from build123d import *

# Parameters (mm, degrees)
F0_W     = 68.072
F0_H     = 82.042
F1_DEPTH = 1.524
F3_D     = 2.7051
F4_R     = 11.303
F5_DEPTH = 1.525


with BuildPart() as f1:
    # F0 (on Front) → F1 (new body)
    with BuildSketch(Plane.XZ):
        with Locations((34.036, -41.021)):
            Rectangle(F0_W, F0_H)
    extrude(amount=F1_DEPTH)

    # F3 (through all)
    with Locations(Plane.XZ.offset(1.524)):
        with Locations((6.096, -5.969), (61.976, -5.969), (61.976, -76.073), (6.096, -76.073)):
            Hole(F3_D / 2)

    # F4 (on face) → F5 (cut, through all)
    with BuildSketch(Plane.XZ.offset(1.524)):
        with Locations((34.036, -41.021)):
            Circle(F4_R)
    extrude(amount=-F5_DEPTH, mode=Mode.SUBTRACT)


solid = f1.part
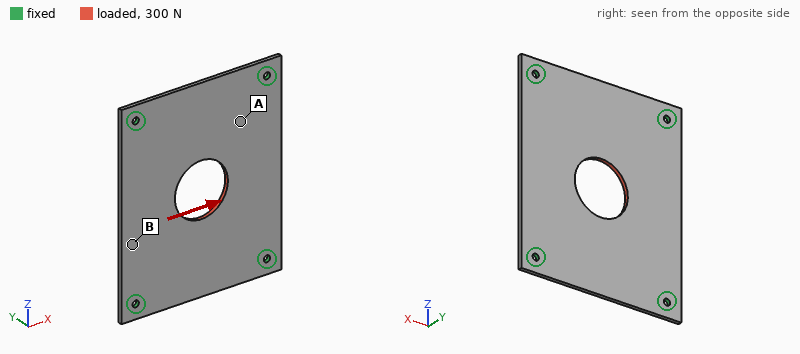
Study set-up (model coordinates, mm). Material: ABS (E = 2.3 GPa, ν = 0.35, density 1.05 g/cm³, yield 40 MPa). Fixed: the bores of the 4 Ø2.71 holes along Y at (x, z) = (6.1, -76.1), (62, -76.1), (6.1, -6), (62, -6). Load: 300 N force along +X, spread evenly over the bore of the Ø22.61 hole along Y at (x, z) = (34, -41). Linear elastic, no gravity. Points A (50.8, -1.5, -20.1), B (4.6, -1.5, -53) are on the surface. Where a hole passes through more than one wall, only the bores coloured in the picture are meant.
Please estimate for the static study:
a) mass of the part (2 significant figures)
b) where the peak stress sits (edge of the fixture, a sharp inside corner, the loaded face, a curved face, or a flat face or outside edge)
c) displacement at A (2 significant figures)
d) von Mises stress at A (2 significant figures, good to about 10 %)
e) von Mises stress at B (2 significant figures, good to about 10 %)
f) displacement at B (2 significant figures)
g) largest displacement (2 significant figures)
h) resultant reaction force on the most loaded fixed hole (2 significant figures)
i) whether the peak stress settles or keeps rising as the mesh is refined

8.3 g
edge of the fixture
44 µm
3.0 MPa
1.5 MPa
63 µm
85 µm
87 N
keeps rising
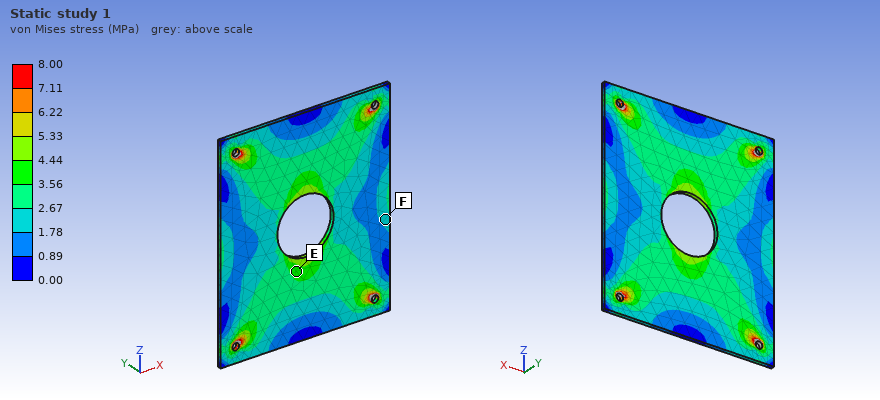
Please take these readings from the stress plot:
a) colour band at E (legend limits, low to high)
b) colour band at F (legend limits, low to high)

3.56 to 4.44 MPa
1.78 to 2.67 MPa
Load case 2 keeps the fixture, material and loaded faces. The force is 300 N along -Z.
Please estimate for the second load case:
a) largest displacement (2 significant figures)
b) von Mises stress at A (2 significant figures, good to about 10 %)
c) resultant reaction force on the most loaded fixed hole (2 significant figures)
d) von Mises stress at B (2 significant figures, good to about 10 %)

61 µm
2.6 MPa
81 N
1.2 MPa
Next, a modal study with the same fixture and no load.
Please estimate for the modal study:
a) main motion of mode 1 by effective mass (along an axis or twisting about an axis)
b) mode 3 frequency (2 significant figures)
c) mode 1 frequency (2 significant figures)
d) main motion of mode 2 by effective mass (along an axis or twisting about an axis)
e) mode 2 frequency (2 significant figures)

along Y
710 Hz
380 Hz
twisting about Z
560 Hz
